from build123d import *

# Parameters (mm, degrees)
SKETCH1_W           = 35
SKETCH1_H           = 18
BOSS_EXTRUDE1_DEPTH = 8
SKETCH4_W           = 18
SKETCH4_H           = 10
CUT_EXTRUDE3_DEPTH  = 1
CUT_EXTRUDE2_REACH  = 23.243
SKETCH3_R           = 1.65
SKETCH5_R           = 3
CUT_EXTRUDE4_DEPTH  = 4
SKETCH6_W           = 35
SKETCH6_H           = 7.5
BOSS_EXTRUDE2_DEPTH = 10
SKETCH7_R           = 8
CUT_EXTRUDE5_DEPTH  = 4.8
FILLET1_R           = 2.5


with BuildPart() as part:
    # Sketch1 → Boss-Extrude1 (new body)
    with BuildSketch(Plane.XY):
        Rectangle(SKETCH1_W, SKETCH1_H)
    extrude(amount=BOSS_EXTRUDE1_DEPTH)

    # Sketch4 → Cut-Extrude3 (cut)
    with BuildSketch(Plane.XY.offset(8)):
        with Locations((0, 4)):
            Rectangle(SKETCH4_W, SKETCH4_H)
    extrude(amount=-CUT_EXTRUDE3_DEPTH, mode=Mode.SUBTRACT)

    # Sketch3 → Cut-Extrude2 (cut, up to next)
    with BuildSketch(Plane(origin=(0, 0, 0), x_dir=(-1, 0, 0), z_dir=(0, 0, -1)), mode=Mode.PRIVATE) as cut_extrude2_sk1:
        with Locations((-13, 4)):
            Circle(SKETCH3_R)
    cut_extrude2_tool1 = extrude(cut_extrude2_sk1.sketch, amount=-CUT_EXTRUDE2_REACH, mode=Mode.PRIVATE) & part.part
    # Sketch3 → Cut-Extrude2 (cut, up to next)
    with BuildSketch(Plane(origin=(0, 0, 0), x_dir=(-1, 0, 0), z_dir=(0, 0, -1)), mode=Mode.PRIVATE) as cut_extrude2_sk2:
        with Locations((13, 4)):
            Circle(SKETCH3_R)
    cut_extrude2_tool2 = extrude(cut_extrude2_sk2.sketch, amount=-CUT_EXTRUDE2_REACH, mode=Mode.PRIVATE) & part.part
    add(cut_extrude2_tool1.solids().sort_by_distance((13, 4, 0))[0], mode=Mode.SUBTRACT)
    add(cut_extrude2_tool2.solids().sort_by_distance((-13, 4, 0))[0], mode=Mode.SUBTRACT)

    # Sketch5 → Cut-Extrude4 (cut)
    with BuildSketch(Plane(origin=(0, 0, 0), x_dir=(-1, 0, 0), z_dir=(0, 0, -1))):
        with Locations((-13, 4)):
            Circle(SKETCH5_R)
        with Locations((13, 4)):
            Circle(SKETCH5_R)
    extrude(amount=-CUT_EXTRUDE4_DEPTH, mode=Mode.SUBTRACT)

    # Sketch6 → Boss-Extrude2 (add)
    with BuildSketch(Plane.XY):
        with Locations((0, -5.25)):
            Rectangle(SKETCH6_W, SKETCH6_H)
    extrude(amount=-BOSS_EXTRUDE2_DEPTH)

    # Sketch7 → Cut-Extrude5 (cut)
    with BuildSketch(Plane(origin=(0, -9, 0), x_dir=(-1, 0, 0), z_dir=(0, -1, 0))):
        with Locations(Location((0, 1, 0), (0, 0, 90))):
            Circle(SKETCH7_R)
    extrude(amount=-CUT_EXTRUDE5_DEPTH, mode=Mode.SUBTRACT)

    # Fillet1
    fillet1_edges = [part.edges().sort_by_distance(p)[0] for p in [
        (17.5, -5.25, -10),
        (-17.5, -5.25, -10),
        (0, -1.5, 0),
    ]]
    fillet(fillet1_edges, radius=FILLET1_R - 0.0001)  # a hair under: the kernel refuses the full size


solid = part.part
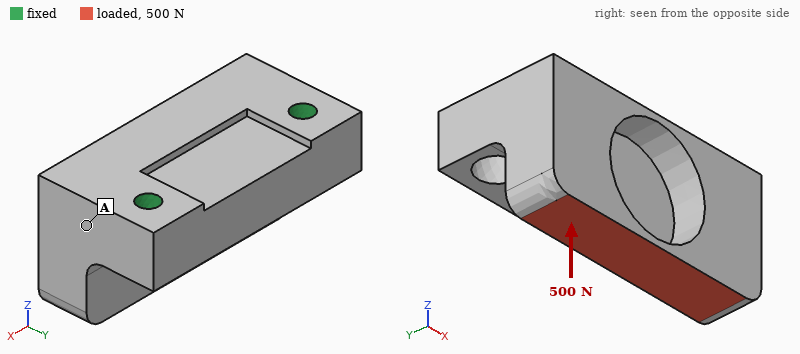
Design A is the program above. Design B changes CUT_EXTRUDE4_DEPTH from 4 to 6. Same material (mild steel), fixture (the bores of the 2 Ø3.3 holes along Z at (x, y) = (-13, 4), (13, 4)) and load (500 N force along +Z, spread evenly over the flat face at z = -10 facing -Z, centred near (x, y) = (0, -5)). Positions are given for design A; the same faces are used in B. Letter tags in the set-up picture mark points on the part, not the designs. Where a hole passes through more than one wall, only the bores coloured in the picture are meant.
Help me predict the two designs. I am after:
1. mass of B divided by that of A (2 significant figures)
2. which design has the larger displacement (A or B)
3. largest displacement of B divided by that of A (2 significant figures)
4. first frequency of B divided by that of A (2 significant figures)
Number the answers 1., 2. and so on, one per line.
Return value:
1. 0.99
2. B
3. 2.5
4. 0.58
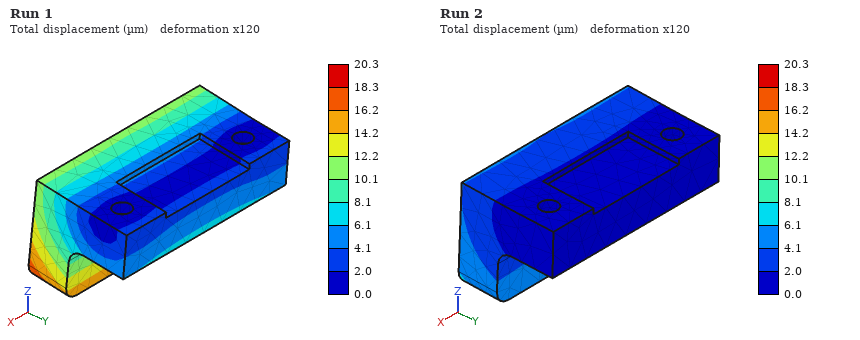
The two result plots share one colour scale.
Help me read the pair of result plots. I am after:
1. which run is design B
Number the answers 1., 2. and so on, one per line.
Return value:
1. Run 1
